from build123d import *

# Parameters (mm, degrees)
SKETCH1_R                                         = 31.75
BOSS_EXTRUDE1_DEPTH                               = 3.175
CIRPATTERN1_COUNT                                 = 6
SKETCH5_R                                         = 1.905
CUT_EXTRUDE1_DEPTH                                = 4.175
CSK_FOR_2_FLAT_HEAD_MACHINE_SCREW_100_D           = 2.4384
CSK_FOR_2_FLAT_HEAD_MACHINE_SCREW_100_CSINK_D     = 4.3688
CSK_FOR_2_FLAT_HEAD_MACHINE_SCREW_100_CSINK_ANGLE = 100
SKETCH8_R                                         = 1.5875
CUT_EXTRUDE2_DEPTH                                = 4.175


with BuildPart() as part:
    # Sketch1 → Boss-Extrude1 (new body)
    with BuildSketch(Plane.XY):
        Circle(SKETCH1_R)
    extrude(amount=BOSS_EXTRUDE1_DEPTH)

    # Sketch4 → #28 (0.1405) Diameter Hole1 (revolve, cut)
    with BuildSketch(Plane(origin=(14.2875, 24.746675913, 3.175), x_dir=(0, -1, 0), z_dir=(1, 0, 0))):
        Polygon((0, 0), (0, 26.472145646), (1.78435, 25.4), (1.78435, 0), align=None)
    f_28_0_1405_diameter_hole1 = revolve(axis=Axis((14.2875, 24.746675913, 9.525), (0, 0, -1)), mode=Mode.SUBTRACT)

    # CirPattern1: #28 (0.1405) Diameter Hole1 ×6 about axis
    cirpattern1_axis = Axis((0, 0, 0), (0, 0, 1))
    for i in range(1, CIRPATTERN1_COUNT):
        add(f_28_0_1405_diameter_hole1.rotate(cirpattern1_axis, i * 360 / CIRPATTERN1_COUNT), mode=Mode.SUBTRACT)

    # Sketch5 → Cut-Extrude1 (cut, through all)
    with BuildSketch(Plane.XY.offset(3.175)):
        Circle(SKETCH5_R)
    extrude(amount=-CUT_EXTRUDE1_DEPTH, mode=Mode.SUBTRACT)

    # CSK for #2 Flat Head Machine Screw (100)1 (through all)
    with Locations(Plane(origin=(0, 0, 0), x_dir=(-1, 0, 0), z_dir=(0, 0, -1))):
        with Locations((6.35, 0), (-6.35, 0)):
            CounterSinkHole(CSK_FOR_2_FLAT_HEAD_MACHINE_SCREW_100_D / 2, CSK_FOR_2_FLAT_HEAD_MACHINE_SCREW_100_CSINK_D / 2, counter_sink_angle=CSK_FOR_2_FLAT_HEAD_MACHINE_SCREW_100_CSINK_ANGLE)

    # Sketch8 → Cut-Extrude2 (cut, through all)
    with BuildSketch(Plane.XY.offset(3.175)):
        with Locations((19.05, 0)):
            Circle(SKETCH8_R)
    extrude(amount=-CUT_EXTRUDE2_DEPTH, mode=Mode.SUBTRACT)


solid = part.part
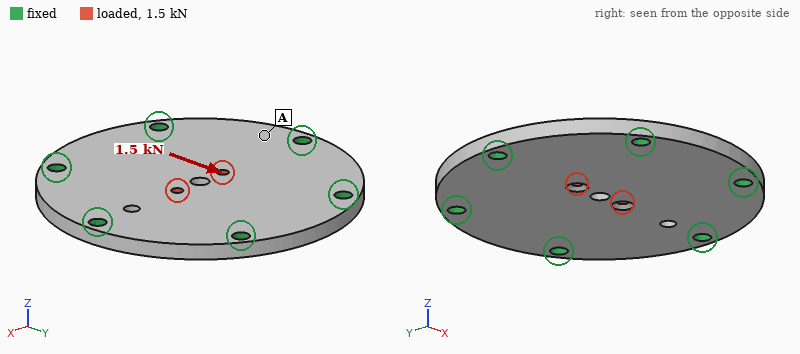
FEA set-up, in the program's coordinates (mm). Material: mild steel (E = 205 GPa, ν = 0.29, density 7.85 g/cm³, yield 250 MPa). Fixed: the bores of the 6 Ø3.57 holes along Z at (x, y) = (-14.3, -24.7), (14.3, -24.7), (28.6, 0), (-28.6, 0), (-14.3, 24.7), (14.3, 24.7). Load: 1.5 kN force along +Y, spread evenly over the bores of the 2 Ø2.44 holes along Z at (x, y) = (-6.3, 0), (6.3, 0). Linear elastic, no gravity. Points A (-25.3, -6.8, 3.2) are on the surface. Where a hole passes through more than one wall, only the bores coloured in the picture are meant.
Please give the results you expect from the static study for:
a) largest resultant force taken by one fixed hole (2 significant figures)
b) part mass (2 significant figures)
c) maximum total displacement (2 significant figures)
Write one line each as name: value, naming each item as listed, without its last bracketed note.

largest resultant force taken by one fixed hole: 320 N
part mass: 77 g
maximum total displacement: 1.6 µm
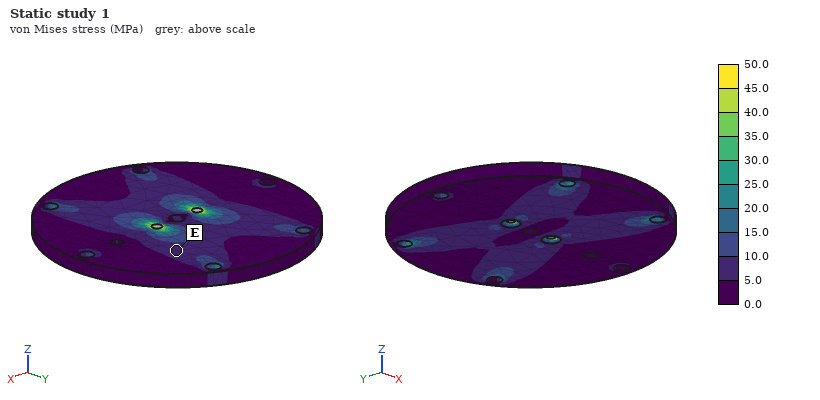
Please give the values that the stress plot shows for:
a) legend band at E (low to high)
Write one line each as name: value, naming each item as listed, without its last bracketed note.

legend band at E: 5.0 to 10.0 MPa
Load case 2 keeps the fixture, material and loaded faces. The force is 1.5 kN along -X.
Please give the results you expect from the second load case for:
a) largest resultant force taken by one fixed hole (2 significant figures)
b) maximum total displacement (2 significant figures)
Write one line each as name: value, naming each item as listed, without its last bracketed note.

largest resultant force taken by one fixed hole: 400 N
maximum total displacement: 1.9 µm
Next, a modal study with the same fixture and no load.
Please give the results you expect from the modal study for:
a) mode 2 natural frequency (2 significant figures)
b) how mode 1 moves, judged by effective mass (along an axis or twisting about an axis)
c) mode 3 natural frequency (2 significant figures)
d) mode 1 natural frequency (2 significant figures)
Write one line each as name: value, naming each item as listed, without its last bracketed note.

mode 2 natural frequency: 16 kHz
how mode 1 moves, judged by effective mass: along Z
mode 3 natural frequency: 16 kHz
mode 1 natural frequency: 8100 Hz
